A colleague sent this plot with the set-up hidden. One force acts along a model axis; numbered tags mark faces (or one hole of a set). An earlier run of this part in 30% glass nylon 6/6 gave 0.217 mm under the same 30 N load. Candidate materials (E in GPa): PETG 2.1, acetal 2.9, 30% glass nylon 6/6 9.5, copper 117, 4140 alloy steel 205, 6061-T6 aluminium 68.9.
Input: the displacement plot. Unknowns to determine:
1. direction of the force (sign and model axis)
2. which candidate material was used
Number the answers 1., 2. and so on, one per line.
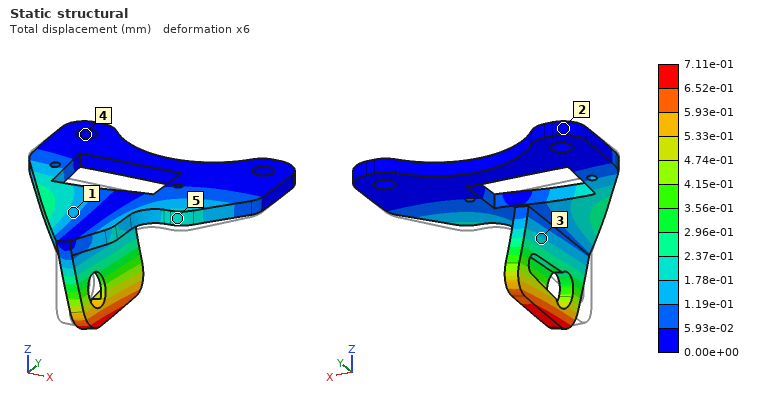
1. +X
2. acetal
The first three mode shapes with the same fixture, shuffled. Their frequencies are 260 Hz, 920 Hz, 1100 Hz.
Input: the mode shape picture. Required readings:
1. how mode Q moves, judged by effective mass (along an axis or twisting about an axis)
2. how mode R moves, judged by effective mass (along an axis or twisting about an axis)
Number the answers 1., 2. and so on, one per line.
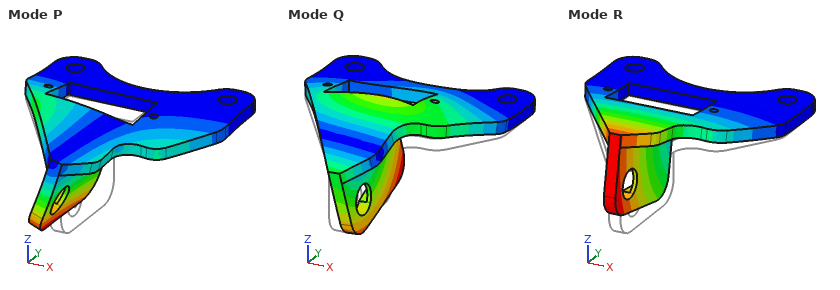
1. along Z
2. along Z
